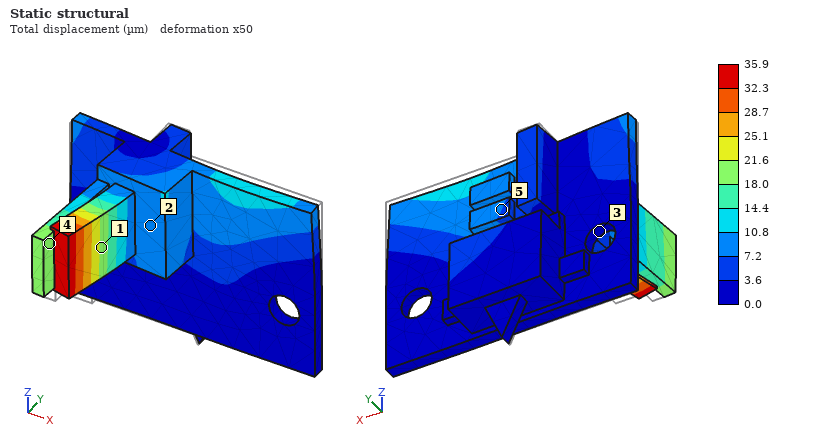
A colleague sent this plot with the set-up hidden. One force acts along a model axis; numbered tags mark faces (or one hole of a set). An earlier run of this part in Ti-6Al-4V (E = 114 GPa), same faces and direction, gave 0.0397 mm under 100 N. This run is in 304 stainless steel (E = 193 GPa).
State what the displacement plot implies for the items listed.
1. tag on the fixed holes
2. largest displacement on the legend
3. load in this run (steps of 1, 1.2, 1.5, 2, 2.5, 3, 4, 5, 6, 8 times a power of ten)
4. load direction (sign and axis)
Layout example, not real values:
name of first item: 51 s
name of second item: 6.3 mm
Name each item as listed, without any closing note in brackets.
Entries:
tag on the fixed holes: 3
largest displacement on the legend: 35.9 µm
load in this run: 150 N
load direction: -X
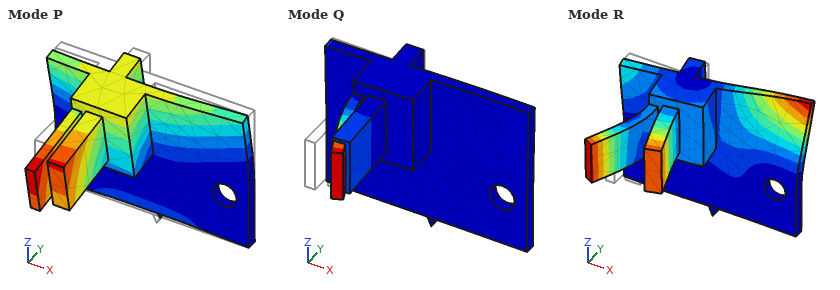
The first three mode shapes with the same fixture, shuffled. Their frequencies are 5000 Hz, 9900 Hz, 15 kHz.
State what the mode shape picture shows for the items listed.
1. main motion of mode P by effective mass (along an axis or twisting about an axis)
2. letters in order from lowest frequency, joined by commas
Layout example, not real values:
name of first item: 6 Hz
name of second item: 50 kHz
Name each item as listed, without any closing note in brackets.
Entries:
main motion of mode P by effective mass: along Y
letters in order from lowest frequency, joined by commas: P, Q, R
